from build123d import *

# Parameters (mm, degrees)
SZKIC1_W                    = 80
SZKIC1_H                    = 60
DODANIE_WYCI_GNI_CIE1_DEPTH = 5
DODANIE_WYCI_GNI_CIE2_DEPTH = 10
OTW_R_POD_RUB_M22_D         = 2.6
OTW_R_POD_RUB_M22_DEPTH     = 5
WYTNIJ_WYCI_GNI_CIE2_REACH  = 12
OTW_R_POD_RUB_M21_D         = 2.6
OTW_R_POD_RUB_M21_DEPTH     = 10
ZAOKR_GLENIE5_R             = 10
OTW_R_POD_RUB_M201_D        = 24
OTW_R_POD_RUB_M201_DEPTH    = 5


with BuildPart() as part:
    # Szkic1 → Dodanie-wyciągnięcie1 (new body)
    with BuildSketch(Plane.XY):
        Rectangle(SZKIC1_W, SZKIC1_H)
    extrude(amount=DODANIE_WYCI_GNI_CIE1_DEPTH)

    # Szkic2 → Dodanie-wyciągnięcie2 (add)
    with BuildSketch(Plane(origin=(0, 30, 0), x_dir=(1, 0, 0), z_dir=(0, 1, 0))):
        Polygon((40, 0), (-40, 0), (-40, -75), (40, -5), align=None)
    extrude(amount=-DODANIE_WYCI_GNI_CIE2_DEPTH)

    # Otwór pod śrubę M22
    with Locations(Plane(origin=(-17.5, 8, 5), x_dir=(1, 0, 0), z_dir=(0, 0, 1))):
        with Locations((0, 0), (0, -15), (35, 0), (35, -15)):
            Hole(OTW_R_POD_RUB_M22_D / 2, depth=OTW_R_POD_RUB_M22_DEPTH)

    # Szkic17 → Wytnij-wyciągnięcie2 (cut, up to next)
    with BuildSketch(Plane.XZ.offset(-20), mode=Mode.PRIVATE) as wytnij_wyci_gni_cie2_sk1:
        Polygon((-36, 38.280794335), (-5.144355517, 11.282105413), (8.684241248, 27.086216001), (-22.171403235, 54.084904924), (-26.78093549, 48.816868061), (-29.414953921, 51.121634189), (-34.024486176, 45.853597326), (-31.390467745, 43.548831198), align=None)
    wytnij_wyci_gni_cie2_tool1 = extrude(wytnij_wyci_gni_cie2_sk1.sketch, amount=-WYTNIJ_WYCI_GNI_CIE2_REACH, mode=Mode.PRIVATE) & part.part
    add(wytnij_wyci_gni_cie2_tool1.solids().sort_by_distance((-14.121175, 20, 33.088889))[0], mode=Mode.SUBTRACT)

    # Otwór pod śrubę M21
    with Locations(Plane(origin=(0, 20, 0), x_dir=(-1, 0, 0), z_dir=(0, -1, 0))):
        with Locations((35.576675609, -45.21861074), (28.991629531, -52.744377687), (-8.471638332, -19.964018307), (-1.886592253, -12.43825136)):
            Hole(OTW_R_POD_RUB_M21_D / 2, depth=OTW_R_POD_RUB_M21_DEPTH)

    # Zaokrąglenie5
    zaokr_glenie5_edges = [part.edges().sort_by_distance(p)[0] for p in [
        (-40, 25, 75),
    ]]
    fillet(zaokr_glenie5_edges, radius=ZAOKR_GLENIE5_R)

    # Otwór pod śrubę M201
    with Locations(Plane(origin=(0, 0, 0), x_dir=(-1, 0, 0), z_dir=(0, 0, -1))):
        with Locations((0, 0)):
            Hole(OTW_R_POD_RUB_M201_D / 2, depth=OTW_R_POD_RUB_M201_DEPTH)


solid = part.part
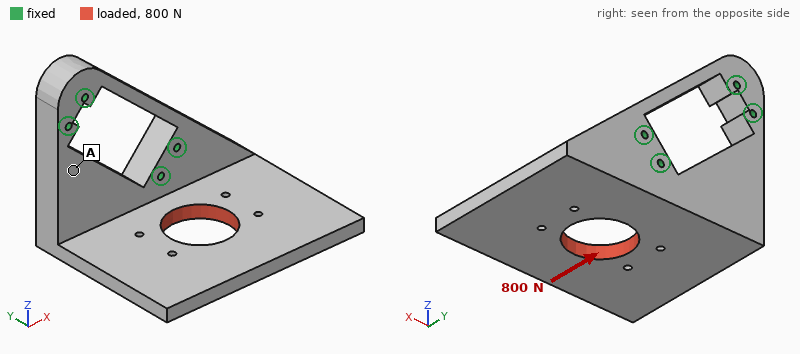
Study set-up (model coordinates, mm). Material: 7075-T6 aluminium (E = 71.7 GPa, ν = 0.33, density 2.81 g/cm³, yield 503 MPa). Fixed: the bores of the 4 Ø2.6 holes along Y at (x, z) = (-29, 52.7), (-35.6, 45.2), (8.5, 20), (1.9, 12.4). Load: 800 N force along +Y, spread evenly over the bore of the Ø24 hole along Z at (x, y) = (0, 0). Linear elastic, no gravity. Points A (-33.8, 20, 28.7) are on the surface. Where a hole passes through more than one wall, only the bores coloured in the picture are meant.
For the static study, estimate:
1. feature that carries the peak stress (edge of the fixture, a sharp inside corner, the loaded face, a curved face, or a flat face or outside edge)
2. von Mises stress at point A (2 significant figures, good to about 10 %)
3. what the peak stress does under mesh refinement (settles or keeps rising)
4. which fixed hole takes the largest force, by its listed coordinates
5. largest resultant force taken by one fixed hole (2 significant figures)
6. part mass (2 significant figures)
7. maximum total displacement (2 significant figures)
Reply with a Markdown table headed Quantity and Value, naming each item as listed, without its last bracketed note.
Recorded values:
| Quantity | Value |
|---|---|
| feature that carries the peak stress | edge of the fixture |
| von Mises stress at point A | 3.4 MPa |
| what the peak stress does under mesh refinement | keeps rising |
| which fixed hole takes the largest force, by its listed coordinates | (1.9, 12.4) |
| largest resultant force taken by one fixed hole | 860 N |
| part mass | 110 g |
| maximum total displacement | 29 µm |
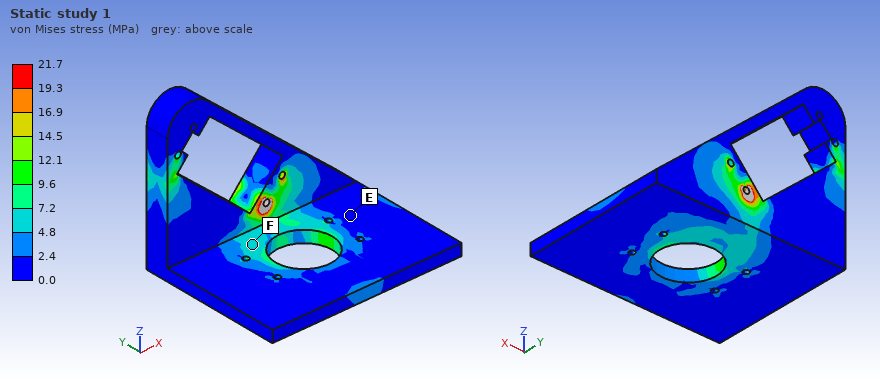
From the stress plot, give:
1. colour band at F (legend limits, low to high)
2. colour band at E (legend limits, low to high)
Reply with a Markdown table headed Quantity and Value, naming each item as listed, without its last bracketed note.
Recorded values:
| Quantity | Value |
|---|---|
| colour band at F | 4.8 to 7.2 MPa |
| colour band at E | 0.0 to 2.4 MPa |
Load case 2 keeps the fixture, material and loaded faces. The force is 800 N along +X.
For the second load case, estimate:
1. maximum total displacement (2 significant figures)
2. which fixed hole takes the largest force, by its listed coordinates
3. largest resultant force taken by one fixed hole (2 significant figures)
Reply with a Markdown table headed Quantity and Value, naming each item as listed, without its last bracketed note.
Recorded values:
| Quantity | Value |
|---|---|
| maximum total displacement | 76 µm |
| which fixed hole takes the largest force, by its listed coordinates | (1.9, 12.4) |
| largest resultant force taken by one fixed hole | 910 N |
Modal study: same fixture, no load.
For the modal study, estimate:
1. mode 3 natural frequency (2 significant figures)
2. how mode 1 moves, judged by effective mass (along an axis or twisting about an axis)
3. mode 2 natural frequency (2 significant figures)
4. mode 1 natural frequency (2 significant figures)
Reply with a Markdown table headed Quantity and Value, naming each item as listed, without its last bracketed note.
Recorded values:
| Quantity | Value |
|---|---|
| mode 3 natural frequency | 2600 Hz |
| how mode 1 moves, judged by effective mass | along Z |
| mode 2 natural frequency | 2100 Hz |
| mode 1 natural frequency | 1200 Hz |
